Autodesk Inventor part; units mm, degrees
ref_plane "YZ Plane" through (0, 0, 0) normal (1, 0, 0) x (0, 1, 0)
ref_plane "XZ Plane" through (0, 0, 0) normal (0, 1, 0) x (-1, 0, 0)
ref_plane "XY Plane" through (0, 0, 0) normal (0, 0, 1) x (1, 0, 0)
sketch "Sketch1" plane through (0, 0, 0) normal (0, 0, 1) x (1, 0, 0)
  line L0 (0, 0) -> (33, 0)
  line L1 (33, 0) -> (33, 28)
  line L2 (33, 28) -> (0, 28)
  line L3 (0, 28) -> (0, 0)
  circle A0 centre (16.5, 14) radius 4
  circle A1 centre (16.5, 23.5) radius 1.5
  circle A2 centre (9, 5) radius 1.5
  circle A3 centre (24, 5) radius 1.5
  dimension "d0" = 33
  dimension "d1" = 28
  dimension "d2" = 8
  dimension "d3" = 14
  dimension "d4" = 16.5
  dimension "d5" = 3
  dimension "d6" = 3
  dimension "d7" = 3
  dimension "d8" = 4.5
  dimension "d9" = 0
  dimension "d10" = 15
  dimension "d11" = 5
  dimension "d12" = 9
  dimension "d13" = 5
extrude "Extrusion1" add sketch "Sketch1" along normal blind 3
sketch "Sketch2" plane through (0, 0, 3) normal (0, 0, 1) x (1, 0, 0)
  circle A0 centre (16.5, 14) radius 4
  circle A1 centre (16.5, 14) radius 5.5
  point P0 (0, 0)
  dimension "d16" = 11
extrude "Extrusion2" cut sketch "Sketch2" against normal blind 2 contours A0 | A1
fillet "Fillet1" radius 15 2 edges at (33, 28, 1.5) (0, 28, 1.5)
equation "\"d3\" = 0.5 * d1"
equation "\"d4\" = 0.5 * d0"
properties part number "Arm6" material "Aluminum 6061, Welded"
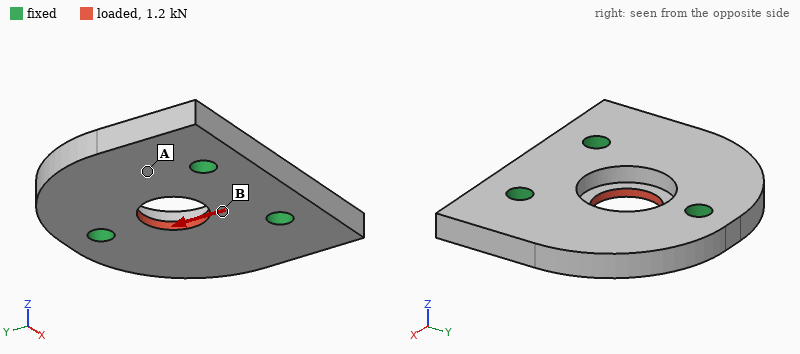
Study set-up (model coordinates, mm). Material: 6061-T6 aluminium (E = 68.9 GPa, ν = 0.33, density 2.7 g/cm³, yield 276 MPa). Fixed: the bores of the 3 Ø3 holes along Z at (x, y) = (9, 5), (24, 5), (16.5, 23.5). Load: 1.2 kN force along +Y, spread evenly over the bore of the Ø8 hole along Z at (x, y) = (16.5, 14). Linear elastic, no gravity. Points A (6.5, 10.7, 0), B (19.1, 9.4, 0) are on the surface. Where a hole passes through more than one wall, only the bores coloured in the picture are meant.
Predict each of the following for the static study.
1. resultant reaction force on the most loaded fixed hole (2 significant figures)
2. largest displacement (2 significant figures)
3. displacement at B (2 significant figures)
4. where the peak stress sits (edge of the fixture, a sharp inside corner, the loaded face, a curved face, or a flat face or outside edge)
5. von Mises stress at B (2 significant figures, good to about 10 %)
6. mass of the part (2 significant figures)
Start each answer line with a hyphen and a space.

- 430 N
- 5.9 µm
- 3.8 µm
- the loaded face
- 42 MPa
- 5.9 g
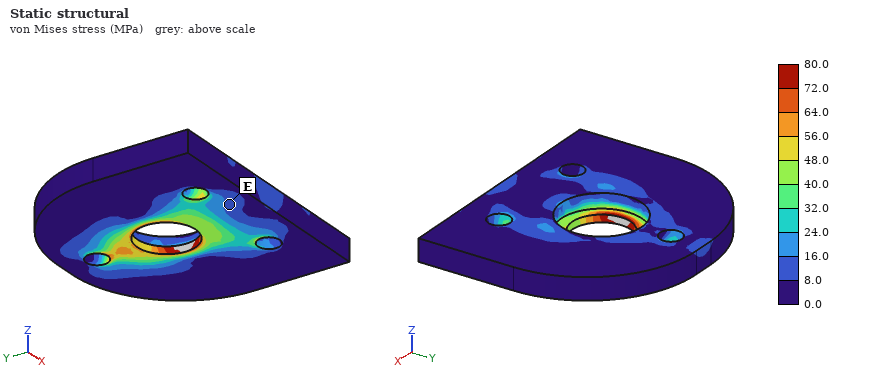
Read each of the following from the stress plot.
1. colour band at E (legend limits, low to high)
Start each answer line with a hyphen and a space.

- 8.0 to 16.0 MPa
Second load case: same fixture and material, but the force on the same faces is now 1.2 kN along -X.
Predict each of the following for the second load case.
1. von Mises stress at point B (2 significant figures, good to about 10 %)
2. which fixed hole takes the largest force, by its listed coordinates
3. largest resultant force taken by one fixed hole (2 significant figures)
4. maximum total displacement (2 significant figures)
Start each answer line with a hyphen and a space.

- 42 MPa
- (16.5, 23.5)
- 560 N
- 6.6 µm
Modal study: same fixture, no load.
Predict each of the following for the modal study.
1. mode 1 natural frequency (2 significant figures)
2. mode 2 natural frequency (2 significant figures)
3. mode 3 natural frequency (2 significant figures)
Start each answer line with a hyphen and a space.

- 16 kHz
- 17 kHz
- 33 kHz
